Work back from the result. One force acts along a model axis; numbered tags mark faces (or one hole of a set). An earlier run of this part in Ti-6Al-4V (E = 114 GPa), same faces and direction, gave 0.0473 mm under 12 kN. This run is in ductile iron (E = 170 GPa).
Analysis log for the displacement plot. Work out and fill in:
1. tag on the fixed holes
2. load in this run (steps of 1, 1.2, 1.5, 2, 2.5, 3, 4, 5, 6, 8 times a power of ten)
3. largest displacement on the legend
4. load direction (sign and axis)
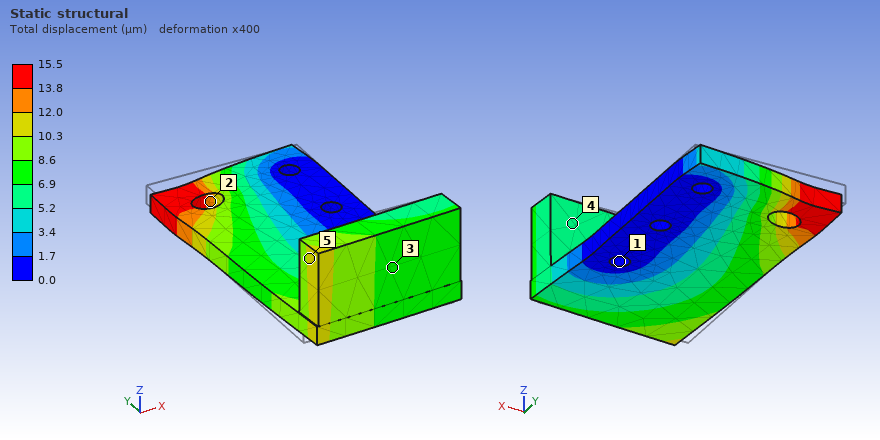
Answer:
1
6 kN
15.5 µm
-Y
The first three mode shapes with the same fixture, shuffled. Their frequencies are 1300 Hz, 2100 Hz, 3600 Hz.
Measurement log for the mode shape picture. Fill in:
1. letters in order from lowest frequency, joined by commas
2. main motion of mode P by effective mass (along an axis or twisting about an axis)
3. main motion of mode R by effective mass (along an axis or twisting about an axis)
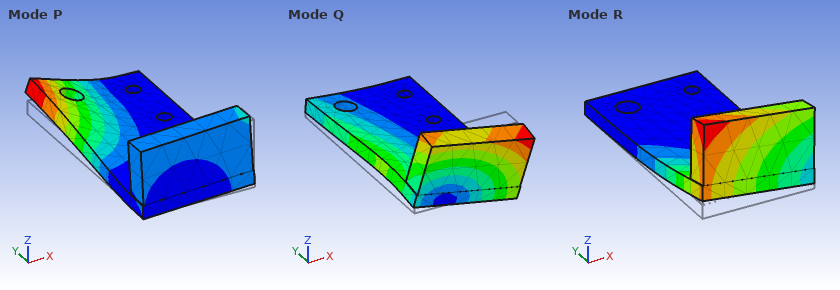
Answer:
R, Q, P
along Z
along Z
